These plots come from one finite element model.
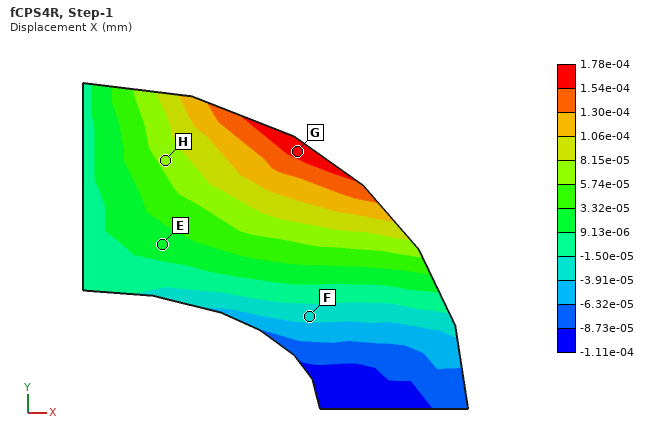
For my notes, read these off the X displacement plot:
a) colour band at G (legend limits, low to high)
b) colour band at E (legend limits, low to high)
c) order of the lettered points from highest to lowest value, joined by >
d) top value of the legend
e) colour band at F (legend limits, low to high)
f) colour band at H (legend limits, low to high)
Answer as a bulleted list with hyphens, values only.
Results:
- 1.54e-04 to 1.78e-04 mm
- 9.13e-06 to 3.32e-05 mm
- G > H > E > F
- 1.78e-04 mm
- -3.91e-05 to -1.50e-05 mm
- 5.74e-05 to 8.15e-05 mm
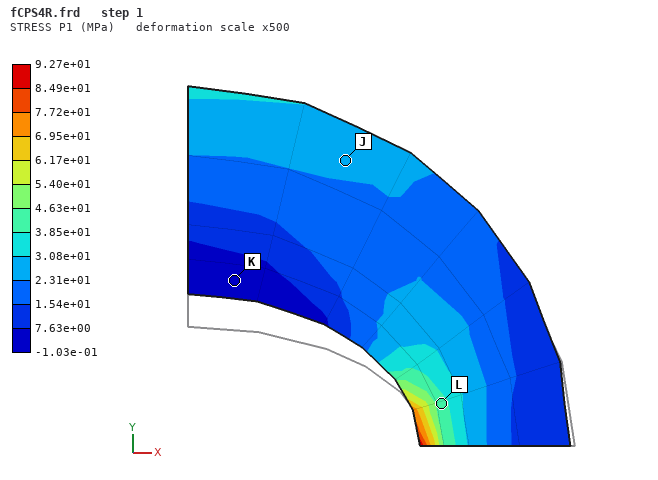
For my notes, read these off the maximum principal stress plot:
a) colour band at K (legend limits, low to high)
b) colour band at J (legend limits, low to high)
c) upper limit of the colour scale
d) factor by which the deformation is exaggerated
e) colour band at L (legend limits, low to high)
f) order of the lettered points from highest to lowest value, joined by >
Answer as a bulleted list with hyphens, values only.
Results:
- -1.03e-01 to 7.63e+00 MPa
- 2.31e+01 to 3.08e+01 MPa
- 9.27e+01 MPa
- 500
- 3.85e+01 to 4.63e+01 MPa
- L > J > K
